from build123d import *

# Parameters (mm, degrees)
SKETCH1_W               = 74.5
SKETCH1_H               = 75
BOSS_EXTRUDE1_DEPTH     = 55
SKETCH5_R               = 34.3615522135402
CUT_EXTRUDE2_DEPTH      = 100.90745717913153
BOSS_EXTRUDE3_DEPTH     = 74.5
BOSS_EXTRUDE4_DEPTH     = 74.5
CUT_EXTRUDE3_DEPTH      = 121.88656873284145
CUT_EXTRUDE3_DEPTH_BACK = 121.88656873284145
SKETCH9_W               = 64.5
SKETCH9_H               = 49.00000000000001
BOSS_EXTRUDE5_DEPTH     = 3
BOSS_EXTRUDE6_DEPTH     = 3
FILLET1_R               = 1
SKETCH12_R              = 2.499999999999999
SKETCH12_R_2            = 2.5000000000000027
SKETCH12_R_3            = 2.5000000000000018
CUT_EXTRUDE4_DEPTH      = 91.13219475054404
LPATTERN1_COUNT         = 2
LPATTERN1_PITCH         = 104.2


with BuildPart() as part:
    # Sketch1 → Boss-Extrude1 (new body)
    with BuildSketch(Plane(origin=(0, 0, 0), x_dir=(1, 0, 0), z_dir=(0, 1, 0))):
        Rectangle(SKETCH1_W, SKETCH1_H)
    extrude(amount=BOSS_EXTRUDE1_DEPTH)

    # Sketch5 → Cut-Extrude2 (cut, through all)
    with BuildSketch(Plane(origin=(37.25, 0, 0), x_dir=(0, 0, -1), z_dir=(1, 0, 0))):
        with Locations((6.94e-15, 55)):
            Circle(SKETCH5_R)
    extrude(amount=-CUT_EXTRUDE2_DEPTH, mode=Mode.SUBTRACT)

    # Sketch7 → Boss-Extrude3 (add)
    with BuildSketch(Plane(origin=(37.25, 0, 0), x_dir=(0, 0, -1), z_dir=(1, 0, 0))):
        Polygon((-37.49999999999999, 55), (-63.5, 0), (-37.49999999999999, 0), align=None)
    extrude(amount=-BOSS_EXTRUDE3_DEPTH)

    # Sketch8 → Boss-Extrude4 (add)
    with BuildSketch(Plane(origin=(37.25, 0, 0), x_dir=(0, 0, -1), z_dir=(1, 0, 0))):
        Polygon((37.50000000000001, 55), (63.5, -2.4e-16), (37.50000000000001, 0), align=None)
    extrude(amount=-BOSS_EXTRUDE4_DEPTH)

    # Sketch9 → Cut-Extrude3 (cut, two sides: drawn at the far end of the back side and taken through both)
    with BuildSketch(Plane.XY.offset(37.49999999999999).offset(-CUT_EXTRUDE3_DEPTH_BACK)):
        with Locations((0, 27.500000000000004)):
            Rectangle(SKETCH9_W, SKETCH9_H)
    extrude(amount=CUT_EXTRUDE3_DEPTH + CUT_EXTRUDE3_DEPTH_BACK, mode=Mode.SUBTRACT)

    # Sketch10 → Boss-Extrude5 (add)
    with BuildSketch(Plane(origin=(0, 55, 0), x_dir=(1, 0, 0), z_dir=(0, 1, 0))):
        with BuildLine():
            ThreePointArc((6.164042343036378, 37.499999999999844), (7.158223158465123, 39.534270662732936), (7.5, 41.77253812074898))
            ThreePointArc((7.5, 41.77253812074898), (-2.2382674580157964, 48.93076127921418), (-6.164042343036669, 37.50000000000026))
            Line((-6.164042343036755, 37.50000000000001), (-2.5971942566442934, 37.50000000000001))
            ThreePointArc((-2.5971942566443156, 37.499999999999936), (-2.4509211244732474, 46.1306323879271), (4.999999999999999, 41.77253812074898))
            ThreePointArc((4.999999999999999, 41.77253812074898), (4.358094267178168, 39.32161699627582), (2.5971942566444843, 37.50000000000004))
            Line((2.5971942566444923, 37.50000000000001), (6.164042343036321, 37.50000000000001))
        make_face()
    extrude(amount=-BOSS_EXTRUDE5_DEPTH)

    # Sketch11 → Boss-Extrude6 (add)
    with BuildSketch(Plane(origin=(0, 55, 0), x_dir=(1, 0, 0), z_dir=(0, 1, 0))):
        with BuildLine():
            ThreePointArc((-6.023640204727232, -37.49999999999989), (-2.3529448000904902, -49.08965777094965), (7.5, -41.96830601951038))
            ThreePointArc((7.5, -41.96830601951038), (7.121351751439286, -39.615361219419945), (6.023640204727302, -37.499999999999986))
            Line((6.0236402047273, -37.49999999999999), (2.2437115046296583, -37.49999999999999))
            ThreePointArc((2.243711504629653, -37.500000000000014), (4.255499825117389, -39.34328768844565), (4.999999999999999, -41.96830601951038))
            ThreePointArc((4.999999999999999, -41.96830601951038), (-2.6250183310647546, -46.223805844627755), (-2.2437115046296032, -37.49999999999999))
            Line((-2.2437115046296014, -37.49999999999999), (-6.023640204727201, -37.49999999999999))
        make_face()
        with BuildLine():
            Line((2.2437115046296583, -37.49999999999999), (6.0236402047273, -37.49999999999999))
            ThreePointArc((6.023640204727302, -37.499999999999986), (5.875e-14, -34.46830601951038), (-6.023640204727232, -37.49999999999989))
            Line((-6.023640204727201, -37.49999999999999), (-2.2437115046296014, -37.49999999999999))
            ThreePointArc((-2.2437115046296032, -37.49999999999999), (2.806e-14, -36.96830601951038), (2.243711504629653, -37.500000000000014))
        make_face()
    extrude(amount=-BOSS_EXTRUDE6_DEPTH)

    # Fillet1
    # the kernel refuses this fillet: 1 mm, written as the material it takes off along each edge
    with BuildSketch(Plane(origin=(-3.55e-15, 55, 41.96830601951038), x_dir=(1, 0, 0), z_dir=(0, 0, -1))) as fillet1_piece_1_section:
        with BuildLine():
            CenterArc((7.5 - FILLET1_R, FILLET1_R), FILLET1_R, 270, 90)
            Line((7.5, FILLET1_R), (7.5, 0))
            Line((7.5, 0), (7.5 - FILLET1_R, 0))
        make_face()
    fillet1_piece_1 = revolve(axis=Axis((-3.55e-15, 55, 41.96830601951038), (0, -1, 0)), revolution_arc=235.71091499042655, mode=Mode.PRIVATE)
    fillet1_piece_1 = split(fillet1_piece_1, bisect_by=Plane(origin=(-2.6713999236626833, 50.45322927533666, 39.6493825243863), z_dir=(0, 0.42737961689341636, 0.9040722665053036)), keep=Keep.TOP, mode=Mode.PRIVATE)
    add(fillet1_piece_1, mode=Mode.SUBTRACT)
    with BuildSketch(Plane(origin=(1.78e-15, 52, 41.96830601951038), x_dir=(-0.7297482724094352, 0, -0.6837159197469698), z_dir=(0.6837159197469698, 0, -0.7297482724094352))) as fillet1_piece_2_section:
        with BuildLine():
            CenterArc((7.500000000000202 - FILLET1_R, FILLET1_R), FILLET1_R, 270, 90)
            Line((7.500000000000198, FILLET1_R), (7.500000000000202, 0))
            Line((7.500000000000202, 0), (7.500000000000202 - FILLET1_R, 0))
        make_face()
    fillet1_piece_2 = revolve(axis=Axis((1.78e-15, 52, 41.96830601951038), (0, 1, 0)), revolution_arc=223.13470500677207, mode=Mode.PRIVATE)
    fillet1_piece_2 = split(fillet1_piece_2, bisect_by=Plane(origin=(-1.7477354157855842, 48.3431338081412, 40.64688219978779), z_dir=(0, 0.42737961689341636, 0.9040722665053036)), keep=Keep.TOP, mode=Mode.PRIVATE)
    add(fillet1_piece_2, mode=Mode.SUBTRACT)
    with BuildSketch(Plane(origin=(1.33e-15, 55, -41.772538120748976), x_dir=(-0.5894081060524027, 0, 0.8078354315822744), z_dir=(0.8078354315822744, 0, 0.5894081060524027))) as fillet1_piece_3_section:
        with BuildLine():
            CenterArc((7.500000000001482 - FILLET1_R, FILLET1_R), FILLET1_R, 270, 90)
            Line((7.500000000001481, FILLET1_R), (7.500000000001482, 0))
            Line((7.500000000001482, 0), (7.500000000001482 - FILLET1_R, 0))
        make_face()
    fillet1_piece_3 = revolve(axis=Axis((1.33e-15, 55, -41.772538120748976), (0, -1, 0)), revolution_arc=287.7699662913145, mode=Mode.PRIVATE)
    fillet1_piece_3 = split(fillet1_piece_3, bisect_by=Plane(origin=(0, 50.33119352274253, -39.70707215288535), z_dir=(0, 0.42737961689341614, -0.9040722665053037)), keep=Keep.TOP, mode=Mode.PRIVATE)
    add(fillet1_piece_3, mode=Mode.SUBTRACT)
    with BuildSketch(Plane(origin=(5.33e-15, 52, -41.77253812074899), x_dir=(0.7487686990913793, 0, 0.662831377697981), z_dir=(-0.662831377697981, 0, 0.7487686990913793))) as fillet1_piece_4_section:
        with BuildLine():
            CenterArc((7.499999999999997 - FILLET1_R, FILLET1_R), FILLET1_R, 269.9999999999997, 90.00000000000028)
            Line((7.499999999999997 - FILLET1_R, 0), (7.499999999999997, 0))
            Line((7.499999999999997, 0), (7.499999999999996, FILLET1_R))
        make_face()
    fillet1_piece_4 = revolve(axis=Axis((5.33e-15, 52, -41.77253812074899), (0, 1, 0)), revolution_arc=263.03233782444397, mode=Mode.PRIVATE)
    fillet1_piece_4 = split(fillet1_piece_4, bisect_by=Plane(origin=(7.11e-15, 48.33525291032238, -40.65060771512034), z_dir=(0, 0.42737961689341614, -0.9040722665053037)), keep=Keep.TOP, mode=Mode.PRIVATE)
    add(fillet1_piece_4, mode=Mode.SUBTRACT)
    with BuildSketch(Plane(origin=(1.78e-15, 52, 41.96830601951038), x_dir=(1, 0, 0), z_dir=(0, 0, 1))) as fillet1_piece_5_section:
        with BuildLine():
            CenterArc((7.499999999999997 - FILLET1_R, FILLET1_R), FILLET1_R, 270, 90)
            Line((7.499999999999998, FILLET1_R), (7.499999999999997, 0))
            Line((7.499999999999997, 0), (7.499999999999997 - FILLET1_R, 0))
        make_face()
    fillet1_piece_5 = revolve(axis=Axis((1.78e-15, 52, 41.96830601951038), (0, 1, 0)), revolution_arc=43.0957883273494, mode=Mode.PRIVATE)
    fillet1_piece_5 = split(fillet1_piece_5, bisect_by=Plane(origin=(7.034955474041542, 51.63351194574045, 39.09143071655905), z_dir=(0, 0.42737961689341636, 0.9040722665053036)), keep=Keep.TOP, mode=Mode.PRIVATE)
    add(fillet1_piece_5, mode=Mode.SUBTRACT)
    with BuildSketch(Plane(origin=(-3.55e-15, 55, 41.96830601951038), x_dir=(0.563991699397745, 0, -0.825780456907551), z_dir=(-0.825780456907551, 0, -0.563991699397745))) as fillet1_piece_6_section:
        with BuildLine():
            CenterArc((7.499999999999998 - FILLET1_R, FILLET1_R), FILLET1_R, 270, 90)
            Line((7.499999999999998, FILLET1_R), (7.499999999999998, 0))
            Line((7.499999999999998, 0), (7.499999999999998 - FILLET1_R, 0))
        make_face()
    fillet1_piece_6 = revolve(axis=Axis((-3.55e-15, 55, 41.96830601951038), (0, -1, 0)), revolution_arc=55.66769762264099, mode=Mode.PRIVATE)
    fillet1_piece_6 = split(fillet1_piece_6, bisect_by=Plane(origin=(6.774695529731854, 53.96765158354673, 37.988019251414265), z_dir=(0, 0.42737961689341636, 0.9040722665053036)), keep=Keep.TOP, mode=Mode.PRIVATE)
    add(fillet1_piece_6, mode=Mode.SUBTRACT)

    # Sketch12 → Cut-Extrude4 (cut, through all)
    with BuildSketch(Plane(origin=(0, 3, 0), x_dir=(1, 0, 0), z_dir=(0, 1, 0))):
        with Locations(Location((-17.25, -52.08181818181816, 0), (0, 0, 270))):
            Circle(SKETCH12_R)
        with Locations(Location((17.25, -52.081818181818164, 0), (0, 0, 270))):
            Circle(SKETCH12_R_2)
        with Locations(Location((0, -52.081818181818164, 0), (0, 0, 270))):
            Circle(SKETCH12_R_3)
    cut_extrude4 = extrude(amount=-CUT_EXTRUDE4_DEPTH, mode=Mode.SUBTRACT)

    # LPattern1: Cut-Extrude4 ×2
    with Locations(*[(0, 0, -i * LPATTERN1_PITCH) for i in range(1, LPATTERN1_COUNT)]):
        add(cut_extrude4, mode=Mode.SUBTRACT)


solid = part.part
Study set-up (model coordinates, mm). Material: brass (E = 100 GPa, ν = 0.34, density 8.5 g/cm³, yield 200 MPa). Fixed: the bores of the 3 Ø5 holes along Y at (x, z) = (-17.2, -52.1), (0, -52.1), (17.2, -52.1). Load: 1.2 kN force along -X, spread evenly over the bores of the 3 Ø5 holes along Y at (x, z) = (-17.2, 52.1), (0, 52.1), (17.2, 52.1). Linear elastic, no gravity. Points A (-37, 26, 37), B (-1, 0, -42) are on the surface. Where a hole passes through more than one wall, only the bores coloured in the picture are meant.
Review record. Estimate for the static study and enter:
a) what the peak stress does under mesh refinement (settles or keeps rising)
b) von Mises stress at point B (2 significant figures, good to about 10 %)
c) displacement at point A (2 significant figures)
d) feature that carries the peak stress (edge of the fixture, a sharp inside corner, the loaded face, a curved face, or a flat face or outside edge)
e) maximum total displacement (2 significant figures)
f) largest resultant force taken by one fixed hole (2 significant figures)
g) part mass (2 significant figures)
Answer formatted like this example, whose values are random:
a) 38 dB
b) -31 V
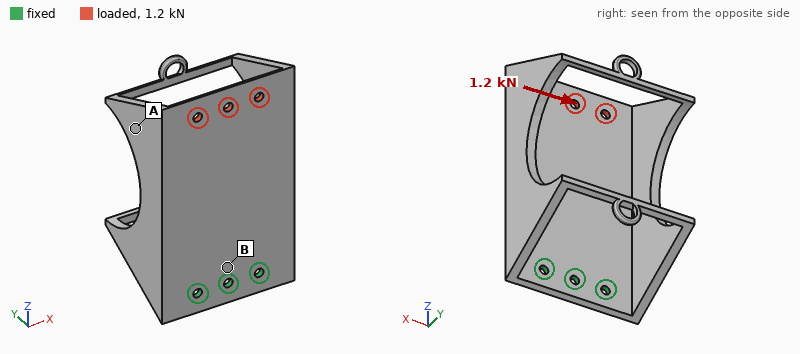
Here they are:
a) keeps rising
b) 33 MPa
c) 0.080 mm
d) edge of the fixture
e) 0.11 mm
f) 3.3 kN
g) 530 g
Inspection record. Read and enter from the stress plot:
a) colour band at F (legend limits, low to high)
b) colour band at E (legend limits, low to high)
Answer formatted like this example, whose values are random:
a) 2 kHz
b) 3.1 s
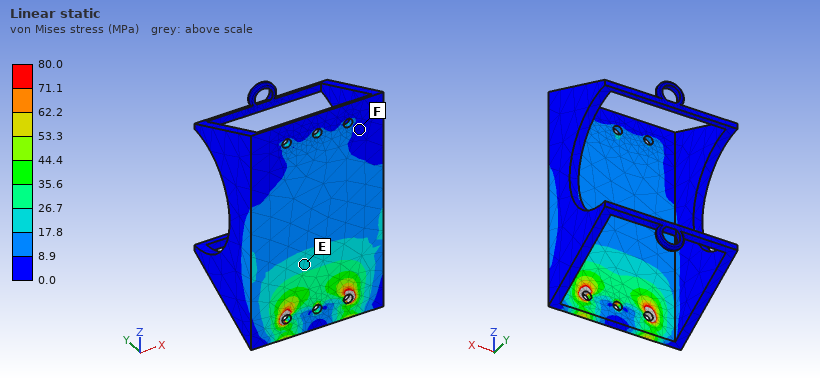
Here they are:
a) 0.0 to 8.9 MPa
b) 17.8 to 26.7 MPa
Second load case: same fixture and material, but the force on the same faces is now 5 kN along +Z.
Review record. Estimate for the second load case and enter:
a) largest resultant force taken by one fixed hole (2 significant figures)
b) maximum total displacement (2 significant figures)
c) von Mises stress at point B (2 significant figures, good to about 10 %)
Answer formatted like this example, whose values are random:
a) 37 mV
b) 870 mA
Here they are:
a) 1.9 kN
b) 53 µm
c) 28 MPa
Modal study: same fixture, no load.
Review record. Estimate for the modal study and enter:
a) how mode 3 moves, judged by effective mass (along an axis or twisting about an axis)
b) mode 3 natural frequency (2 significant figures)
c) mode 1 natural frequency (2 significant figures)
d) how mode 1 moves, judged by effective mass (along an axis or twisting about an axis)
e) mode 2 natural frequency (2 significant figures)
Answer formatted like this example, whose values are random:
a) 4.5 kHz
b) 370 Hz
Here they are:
a) along X
b) 820 Hz
c) 160 Hz
d) along Y
e) 270 Hz
